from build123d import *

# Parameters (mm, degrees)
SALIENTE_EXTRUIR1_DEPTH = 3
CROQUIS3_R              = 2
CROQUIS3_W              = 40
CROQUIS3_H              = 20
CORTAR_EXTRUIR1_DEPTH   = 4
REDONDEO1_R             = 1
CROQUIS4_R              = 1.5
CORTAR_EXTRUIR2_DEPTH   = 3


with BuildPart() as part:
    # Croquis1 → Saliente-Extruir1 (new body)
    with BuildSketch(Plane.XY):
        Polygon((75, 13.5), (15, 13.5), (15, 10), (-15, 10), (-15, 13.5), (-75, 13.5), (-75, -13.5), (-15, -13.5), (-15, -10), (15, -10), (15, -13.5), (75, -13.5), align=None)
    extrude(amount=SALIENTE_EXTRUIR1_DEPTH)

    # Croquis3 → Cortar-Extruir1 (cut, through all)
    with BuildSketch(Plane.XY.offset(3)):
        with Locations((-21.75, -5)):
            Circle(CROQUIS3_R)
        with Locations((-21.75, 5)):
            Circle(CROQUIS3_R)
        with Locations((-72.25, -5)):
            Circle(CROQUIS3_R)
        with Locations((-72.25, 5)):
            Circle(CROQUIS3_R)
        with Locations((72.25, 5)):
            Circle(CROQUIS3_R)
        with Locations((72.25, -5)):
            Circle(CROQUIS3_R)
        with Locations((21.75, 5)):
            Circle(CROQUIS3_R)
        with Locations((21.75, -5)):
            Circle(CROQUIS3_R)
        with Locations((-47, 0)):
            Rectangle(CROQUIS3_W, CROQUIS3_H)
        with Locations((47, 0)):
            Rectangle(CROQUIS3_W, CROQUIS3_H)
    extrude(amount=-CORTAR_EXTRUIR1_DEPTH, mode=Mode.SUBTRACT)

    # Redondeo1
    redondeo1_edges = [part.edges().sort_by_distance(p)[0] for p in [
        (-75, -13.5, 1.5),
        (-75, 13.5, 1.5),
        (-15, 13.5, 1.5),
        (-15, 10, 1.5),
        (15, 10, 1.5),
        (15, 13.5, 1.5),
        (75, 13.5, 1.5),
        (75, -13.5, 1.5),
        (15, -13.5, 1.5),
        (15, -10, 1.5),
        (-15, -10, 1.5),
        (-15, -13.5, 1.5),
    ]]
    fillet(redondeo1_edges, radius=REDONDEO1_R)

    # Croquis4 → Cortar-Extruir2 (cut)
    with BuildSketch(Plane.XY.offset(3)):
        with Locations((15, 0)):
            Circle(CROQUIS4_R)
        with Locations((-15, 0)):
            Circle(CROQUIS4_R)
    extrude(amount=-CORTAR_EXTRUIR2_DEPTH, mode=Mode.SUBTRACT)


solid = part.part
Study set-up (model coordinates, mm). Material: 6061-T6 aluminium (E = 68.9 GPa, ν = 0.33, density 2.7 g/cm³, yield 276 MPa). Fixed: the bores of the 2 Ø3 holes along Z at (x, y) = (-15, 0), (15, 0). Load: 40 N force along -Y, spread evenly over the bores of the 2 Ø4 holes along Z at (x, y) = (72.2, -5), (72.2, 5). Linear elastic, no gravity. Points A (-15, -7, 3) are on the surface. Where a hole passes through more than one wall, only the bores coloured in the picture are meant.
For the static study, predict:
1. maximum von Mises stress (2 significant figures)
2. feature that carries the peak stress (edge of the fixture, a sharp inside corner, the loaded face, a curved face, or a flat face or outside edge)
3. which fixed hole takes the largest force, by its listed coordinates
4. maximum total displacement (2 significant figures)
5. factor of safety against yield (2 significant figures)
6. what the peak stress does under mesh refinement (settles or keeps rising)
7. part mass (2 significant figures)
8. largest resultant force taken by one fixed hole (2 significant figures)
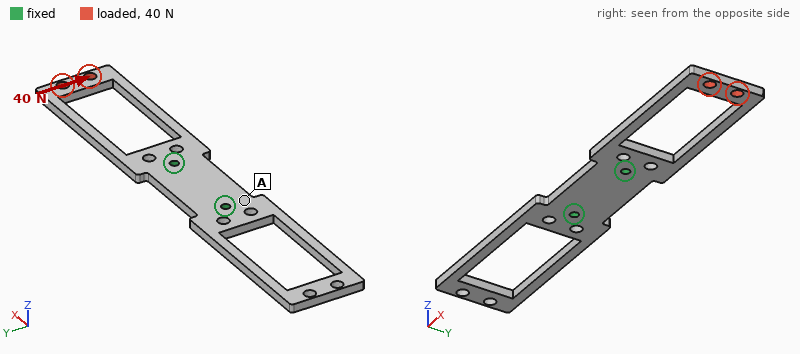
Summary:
65 MPa
a flat face or outside edge
(15, 0)
0.23 mm
4.2
settles
17 g
100 N
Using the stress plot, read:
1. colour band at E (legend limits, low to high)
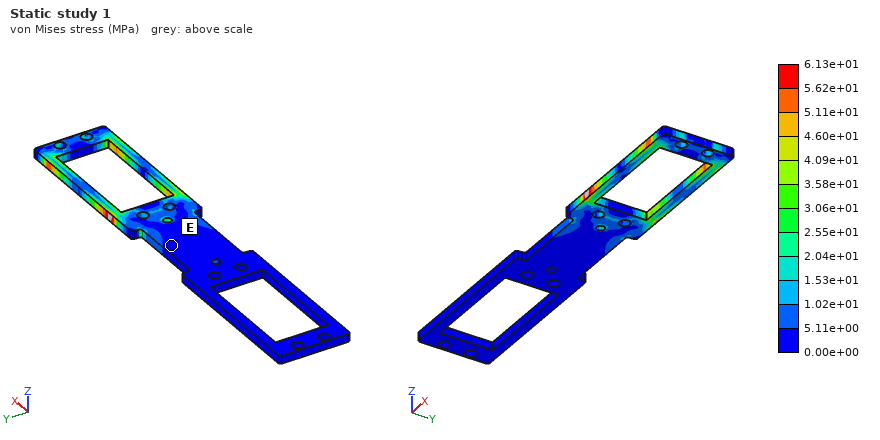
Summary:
0.00e+00 to 5.11e+00 MPa
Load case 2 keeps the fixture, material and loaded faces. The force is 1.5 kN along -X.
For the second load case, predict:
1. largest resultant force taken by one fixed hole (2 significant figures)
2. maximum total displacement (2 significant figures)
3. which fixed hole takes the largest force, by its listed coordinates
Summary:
1.1 kN
0.12 mm
(15, 0)
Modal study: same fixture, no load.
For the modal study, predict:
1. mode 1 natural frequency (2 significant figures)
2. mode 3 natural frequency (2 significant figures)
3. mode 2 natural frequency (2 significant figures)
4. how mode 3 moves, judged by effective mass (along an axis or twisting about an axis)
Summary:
550 Hz
1400 Hz
560 Hz
along Y
